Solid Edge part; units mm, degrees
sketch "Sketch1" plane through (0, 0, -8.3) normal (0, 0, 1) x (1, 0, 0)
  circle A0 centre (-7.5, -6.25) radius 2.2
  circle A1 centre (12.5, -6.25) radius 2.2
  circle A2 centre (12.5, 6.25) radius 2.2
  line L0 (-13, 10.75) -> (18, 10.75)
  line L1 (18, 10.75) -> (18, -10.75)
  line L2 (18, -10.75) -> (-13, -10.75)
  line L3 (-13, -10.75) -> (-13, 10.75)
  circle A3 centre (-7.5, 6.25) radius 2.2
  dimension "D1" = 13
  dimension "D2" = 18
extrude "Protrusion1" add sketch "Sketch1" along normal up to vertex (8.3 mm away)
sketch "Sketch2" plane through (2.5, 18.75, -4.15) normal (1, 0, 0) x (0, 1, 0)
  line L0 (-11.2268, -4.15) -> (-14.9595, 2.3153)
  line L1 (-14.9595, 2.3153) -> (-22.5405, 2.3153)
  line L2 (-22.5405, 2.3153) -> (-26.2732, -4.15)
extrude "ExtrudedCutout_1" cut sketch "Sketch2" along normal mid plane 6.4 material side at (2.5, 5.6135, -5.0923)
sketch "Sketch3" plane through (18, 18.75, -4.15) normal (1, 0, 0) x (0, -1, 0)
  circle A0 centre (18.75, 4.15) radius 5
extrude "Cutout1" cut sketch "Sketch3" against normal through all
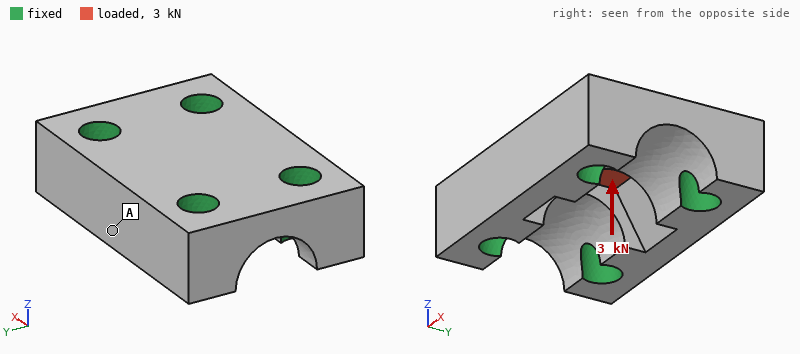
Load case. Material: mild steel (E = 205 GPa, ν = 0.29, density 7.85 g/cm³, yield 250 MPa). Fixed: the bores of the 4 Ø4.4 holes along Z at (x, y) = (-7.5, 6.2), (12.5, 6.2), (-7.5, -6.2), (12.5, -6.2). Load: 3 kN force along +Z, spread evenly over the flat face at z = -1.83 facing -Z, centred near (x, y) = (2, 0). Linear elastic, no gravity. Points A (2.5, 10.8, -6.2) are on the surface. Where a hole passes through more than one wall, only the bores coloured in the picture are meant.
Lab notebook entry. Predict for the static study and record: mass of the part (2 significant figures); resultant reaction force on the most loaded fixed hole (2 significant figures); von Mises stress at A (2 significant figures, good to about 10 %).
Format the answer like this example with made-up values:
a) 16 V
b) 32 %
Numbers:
a) 28 g
b) 880 N
c) 23 MPa
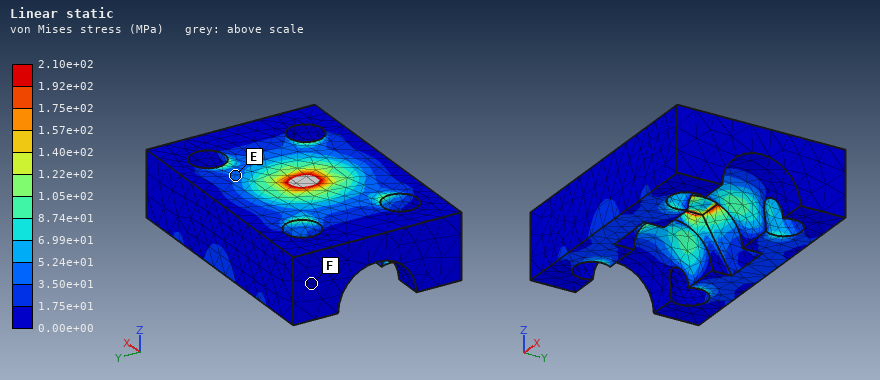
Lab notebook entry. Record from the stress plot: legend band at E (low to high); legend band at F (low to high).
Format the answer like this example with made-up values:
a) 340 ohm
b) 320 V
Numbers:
a) 3.50e+01 to 5.24e+01 MPa
b) 0.00e+00 to 1.75e+01 MPa
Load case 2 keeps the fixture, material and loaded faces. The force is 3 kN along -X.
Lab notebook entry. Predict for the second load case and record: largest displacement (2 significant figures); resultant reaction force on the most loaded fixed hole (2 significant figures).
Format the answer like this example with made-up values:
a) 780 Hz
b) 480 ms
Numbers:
a) 3.3 µm
b) 800 N
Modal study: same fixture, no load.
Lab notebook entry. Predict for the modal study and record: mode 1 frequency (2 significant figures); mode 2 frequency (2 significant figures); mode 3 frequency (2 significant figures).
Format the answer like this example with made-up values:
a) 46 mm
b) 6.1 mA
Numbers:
a) 74 kHz
b) 75 kHz
c) 80 kHz
